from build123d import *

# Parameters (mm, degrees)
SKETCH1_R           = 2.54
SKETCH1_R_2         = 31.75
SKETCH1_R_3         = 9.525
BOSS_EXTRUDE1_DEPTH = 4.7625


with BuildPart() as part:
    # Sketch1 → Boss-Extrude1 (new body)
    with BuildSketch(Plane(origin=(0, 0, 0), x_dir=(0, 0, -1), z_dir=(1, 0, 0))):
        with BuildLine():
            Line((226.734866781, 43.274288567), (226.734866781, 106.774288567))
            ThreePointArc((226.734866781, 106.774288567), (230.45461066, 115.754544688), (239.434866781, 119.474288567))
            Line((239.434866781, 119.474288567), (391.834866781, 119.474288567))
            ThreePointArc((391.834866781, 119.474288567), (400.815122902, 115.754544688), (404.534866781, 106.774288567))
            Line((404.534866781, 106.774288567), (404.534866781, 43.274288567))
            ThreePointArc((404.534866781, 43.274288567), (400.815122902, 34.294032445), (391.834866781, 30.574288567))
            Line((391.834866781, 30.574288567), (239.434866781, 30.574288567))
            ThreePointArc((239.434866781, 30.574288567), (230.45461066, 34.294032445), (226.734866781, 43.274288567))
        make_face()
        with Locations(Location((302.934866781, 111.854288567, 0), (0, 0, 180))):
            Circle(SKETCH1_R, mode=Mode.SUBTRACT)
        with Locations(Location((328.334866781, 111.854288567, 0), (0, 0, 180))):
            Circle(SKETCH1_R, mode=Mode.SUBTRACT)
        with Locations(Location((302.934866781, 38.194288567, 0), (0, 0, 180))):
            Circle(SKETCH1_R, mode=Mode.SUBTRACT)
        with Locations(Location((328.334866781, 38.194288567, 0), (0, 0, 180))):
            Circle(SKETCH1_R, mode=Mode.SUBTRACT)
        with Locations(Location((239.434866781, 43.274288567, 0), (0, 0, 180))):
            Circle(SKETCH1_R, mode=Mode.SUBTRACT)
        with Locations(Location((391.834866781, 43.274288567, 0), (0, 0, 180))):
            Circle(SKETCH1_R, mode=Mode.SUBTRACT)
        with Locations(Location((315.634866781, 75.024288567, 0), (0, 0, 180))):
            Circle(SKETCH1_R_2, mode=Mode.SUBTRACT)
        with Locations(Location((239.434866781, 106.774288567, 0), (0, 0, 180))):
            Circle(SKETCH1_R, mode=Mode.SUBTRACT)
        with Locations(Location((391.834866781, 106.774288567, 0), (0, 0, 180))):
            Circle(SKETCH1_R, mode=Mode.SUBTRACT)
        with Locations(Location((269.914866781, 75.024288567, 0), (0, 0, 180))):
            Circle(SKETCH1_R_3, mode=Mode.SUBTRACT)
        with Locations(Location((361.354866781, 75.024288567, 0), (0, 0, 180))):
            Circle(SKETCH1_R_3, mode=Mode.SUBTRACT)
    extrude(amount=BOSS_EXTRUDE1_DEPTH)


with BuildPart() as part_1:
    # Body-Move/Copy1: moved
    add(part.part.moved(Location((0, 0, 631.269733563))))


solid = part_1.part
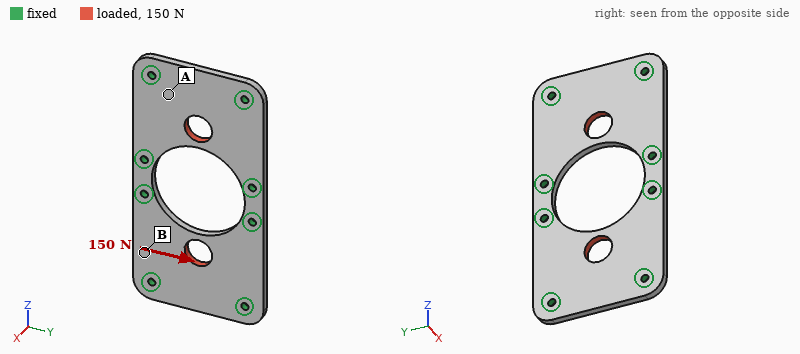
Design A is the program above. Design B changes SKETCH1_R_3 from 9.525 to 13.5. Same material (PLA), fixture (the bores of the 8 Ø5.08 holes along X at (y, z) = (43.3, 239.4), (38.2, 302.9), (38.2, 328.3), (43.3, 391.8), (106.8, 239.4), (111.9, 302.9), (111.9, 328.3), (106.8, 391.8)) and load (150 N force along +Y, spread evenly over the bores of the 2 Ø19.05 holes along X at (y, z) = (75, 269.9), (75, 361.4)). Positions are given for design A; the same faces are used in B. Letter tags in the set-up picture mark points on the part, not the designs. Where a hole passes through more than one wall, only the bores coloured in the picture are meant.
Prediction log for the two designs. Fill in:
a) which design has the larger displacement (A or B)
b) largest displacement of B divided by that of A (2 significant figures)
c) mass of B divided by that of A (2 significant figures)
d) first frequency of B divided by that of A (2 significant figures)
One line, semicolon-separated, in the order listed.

B; 1.2; 0.95; 1.1
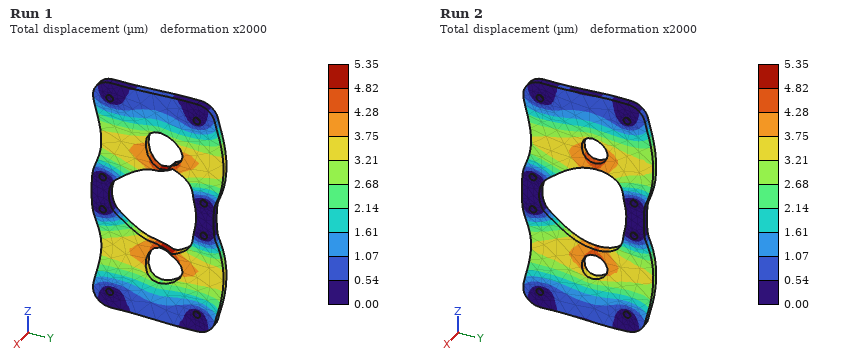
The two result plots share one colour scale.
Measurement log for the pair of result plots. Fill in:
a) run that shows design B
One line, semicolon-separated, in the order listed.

Run 1
